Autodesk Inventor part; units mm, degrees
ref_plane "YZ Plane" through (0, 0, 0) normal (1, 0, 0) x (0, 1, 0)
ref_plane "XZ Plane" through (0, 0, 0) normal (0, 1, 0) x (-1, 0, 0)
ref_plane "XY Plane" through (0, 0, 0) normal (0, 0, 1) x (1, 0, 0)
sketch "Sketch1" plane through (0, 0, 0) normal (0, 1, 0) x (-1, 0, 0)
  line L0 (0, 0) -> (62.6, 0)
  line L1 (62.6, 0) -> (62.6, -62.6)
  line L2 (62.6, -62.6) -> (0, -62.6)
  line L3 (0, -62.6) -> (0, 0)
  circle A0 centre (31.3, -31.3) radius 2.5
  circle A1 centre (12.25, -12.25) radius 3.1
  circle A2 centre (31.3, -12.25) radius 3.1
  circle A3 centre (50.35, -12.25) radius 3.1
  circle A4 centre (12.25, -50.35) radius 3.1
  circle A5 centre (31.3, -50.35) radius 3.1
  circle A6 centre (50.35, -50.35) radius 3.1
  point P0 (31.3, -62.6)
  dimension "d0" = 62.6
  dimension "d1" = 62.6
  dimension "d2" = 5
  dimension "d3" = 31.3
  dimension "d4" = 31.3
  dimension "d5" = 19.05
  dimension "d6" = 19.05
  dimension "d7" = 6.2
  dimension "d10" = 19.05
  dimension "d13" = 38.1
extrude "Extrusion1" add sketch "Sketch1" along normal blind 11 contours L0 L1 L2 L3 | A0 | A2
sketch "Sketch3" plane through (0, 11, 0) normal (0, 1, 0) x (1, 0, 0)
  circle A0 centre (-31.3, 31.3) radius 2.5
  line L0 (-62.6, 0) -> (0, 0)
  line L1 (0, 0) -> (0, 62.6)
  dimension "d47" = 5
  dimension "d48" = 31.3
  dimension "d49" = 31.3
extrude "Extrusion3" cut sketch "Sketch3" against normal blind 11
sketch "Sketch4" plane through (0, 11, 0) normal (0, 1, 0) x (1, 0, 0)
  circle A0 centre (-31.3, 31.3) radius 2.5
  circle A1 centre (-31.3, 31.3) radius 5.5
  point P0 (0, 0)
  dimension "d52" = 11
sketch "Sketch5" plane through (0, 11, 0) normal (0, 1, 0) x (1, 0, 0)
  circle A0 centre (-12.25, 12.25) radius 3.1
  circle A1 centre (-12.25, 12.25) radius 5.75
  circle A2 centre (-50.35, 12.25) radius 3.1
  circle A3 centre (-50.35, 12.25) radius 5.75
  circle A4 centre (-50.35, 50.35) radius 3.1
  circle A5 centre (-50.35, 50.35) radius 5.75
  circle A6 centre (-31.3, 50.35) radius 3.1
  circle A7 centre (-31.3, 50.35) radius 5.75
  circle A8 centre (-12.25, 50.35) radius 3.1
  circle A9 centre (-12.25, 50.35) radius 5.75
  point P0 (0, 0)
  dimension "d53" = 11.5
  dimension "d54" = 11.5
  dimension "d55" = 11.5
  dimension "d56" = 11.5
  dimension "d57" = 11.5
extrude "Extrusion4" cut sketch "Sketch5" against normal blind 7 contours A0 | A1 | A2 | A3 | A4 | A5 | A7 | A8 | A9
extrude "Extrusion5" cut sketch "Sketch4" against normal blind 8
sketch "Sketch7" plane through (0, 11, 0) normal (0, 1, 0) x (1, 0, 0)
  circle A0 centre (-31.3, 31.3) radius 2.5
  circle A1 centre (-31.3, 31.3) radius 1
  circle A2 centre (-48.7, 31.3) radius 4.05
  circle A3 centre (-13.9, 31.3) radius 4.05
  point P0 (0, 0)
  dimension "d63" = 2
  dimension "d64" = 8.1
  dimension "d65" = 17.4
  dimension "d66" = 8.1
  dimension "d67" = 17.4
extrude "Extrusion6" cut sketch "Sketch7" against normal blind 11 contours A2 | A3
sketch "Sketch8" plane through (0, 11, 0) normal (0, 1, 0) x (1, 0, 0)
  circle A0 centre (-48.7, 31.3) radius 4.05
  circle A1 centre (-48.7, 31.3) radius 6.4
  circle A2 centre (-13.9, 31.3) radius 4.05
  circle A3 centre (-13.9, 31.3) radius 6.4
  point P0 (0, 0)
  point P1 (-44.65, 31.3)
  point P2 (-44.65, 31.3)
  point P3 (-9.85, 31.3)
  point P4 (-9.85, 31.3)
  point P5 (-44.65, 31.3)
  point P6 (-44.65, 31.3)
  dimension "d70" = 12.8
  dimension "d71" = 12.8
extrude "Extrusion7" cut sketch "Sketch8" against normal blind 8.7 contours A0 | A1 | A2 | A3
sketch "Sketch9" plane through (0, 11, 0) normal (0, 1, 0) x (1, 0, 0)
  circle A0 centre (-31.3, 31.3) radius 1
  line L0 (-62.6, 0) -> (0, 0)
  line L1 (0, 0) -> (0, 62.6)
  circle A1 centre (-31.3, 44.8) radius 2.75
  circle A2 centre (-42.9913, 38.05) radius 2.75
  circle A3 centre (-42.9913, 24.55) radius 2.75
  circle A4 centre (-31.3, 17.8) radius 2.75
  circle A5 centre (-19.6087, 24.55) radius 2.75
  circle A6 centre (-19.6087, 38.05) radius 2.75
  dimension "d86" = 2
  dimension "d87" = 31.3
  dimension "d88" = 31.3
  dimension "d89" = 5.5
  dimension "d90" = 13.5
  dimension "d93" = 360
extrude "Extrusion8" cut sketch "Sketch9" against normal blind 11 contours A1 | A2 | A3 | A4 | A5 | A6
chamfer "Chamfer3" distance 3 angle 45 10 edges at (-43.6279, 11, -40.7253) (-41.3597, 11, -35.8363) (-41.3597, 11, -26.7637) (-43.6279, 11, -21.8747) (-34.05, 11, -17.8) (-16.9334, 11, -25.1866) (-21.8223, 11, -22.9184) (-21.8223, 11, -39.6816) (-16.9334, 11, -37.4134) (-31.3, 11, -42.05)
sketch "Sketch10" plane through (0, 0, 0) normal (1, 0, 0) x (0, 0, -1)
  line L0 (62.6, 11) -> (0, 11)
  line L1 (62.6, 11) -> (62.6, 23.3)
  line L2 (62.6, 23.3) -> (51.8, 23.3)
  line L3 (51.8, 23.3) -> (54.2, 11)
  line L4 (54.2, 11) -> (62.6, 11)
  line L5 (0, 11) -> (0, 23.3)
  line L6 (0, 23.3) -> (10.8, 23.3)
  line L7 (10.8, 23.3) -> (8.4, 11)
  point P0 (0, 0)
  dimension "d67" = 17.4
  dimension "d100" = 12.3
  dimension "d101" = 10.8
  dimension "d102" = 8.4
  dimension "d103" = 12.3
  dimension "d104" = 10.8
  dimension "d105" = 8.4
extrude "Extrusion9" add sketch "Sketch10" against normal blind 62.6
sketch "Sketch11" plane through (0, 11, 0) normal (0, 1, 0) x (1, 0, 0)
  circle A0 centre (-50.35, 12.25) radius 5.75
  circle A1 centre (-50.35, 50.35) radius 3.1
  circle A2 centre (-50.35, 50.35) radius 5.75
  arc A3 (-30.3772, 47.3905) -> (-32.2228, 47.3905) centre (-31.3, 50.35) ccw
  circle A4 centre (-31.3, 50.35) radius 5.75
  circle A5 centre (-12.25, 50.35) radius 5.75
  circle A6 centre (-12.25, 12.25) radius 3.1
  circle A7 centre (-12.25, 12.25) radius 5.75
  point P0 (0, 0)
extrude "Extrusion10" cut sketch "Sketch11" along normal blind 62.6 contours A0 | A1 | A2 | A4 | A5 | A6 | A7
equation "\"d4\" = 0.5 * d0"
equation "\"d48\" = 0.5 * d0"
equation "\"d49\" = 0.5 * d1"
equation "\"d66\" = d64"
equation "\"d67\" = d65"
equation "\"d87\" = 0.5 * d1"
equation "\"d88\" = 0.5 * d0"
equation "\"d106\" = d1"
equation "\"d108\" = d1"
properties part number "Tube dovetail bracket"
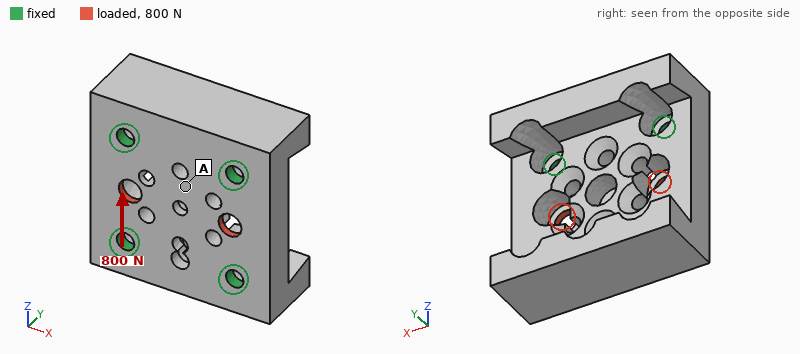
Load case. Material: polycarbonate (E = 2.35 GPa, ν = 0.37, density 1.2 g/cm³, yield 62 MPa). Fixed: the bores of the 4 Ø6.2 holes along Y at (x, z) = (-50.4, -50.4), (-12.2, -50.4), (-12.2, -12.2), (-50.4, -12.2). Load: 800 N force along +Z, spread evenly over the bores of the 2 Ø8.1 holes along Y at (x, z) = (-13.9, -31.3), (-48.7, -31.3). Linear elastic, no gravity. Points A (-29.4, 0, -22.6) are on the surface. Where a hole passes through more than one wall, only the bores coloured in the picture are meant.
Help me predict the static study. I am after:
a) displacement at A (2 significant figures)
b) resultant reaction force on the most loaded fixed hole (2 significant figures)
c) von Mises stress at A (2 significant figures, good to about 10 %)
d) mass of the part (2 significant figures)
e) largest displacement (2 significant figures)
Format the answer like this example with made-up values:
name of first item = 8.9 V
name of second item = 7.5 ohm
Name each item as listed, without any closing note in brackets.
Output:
displacement at A = 9.8 µm
resultant reaction force on the most loaded fixed hole = 200 N
von Mises stress at A = 1.0 MPa
mass of the part = 56 g
largest displacement = 41 µm
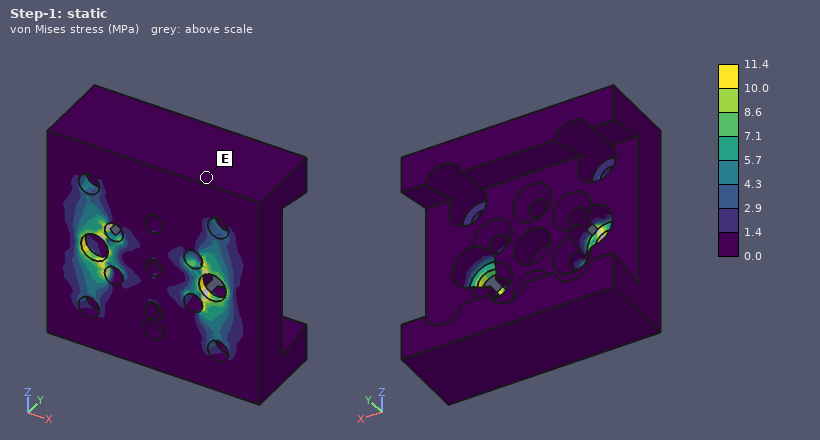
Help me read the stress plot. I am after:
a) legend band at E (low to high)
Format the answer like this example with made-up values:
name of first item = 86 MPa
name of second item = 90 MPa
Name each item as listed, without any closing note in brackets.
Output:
legend band at E = 0.0 to 1.4 MPa
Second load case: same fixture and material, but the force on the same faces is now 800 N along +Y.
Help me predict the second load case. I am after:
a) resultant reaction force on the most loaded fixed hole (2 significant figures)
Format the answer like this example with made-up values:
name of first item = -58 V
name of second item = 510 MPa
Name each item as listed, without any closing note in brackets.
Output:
resultant reaction force on the most loaded fixed hole = 230 N
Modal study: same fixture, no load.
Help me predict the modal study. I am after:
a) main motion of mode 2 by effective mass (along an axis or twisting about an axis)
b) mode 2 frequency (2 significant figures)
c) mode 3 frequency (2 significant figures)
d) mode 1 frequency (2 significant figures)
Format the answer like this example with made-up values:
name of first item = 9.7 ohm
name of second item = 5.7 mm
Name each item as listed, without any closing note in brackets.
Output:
main motion of mode 2 by effective mass = along Z
mode 2 frequency = 2600 Hz
mode 3 frequency = 3400 Hz
mode 1 frequency = 2500 Hz
